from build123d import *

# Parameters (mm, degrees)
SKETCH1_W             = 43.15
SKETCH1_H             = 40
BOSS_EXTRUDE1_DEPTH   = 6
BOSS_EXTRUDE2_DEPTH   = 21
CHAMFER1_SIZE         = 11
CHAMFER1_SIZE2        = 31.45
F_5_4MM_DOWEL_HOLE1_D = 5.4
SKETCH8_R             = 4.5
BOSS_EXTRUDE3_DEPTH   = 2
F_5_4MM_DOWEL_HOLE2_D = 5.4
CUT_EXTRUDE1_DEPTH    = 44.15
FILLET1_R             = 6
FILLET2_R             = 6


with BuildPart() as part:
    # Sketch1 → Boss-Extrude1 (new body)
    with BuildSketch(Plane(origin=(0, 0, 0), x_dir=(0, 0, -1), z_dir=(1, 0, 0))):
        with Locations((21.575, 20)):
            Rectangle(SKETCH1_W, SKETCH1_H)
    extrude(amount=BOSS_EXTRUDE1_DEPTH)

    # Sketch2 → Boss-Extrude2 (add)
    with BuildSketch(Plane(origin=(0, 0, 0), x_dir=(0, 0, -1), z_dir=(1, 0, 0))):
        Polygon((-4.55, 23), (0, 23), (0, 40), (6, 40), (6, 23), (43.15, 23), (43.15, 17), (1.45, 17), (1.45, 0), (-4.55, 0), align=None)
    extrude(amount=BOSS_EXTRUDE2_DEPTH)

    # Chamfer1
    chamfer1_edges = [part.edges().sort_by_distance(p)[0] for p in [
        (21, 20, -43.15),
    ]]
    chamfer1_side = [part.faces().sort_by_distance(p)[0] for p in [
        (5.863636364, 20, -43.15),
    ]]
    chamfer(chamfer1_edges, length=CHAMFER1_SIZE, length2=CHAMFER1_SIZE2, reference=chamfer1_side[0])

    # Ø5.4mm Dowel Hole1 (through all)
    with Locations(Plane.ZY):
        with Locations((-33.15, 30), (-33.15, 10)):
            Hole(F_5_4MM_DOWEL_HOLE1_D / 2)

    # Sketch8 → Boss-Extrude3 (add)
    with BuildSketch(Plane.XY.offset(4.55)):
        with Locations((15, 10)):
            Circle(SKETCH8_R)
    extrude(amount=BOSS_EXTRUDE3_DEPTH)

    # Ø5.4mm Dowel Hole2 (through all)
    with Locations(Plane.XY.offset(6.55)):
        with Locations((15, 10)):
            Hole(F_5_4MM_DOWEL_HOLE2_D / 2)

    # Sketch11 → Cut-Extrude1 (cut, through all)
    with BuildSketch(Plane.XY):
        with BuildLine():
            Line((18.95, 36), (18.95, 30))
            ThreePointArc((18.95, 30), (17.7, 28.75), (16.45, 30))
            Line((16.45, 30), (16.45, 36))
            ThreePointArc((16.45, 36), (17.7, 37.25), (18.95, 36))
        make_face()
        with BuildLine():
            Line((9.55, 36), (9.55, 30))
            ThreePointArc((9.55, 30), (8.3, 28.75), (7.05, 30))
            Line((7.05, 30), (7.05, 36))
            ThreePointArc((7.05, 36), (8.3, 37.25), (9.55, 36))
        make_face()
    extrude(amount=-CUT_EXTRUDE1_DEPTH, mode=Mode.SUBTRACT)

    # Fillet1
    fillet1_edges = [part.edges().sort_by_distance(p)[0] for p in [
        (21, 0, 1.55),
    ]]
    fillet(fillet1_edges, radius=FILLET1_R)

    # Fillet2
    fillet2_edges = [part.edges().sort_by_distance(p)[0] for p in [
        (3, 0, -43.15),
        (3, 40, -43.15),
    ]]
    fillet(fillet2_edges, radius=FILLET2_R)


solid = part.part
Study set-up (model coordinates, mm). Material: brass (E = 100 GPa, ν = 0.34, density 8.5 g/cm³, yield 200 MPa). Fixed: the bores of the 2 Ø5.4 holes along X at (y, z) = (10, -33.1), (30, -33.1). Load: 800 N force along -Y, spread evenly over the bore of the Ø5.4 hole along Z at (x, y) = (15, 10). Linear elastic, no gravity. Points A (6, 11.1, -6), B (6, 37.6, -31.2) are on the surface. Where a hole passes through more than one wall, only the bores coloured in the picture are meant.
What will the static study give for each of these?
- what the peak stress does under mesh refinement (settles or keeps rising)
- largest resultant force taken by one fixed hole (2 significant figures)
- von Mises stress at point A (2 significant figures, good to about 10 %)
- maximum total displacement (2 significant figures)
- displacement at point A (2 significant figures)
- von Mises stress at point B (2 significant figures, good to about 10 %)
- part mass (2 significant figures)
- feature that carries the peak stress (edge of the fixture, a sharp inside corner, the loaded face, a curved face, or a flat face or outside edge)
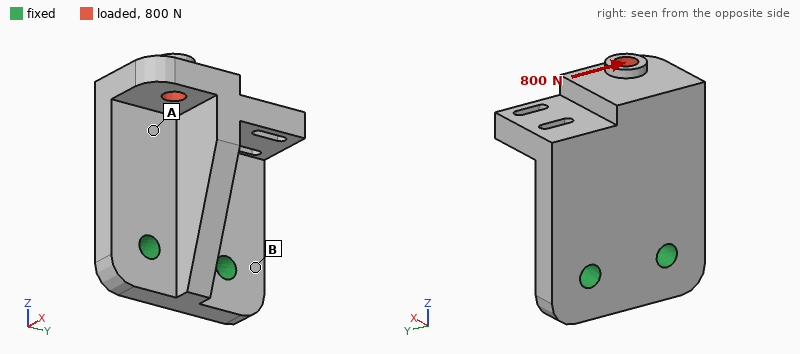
keeps rising
1.3 kN
21 MPa
38 µm
13 µm
8.2 MPa
140 g
edge of the fixture
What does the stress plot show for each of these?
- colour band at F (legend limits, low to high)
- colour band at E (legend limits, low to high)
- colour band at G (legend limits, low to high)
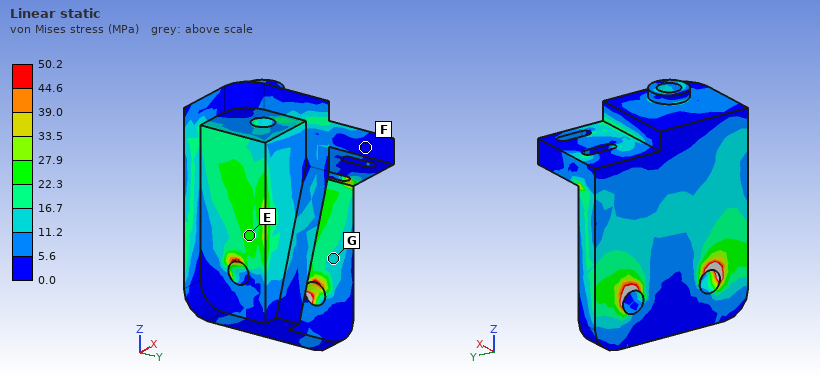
0.0 to 5.6 MPa
22.3 to 27.9 MPa
11.2 to 16.7 MPa
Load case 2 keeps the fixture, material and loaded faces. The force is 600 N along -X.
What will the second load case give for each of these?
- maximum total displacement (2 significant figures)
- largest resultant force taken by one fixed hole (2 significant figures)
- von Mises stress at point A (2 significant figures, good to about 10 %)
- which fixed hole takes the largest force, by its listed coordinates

83 µm
580 N
17 MPa
(10, -33.1)
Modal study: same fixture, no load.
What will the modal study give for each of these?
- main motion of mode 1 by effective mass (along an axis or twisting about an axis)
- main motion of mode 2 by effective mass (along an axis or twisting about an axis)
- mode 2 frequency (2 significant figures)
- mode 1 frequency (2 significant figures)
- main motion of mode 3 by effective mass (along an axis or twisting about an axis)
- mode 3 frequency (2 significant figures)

along X
along Y
3800 Hz
2200 Hz
along Y
6900 Hz
